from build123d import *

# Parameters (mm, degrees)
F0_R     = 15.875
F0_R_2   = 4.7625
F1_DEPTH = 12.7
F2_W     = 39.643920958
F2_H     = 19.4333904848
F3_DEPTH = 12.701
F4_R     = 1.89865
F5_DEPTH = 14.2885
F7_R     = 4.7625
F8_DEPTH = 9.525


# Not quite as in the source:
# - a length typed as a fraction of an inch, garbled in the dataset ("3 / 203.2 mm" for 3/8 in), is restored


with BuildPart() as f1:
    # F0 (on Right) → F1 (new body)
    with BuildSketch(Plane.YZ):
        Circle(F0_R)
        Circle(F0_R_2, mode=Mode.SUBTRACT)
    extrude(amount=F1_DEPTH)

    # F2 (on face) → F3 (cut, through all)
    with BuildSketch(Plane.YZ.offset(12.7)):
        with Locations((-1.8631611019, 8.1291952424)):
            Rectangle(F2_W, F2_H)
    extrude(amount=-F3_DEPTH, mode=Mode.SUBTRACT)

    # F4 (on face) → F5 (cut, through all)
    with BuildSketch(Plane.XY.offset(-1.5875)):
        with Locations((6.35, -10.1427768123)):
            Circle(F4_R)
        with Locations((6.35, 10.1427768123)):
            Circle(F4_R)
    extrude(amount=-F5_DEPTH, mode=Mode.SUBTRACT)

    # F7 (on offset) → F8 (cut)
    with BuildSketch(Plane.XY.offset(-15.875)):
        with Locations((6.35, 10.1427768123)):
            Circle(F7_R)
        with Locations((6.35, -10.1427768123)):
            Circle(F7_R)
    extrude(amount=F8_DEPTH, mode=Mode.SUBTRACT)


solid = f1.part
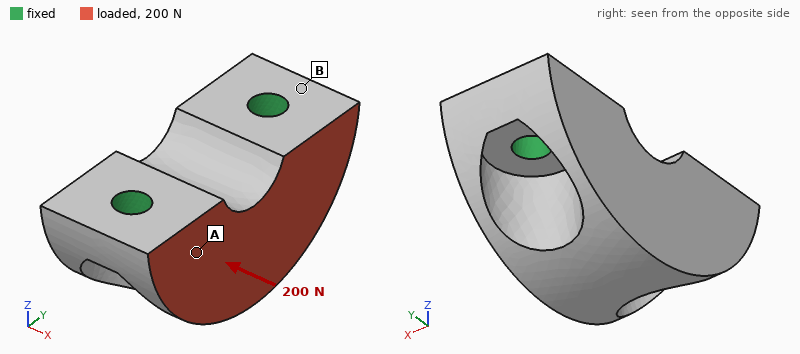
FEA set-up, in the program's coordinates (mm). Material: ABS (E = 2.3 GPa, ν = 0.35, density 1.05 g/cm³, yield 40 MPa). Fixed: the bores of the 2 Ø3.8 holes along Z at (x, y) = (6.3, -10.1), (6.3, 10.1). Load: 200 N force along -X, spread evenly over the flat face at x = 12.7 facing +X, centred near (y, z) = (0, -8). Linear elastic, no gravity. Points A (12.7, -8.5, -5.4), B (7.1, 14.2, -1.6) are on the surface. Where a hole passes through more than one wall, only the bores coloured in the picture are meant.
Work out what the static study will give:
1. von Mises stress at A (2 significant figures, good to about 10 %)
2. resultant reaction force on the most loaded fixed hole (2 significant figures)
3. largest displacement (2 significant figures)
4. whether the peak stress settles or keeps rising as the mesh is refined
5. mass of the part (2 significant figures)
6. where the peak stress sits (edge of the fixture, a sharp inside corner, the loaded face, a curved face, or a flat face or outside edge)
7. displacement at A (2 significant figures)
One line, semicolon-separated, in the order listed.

4.4 MPa; 100 N; 65 µm; keeps rising; 3.4 g; edge of the fixture; 21 µm
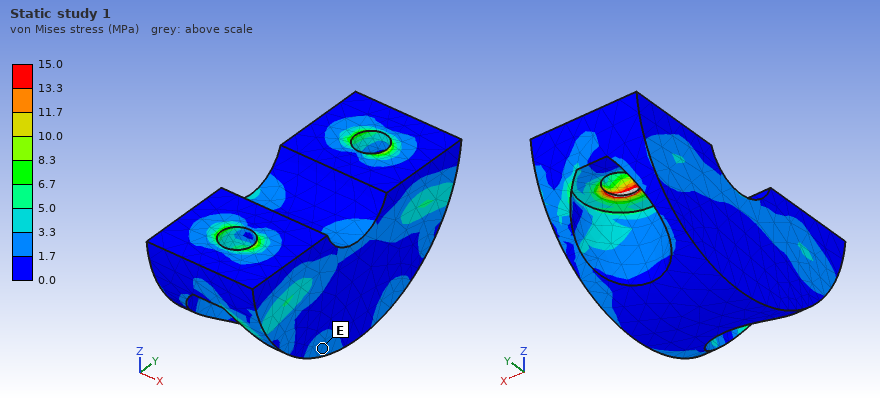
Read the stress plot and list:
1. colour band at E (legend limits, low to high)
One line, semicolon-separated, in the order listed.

1.7 to 3.3 MPa
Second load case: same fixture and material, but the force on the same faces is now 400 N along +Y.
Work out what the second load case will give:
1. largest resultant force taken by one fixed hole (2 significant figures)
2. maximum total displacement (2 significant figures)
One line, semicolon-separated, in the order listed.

230 N; 56 µm
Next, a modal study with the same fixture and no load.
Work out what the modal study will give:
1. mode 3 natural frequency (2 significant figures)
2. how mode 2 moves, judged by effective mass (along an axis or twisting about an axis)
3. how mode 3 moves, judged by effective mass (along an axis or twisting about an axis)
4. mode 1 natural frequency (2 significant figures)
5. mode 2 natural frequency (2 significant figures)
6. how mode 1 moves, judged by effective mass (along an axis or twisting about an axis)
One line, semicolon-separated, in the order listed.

13 kHz; along Z; along Y; 5700 Hz; 12 kHz; along X
